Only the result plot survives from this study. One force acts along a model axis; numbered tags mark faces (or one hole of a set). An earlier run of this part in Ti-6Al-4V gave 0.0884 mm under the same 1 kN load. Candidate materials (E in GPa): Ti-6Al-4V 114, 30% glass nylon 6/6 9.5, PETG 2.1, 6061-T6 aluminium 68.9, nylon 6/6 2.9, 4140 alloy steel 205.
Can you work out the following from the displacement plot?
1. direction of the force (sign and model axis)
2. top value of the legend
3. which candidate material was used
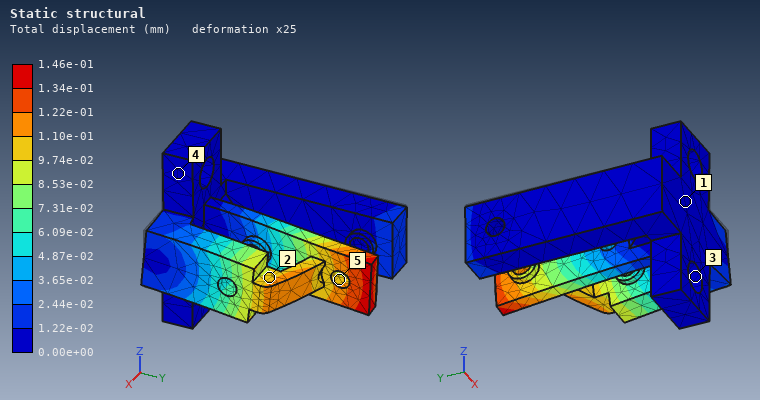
-Z
1.46e-01 mm
6061-T6 aluminium
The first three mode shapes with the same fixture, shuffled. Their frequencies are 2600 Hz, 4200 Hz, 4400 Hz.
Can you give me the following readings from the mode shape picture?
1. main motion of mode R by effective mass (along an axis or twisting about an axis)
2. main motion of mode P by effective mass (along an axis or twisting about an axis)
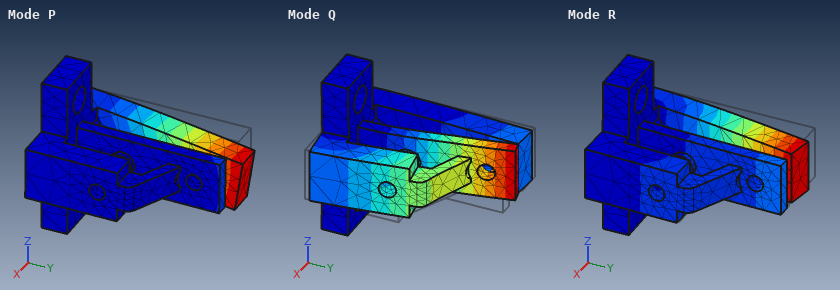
along X
along Z
